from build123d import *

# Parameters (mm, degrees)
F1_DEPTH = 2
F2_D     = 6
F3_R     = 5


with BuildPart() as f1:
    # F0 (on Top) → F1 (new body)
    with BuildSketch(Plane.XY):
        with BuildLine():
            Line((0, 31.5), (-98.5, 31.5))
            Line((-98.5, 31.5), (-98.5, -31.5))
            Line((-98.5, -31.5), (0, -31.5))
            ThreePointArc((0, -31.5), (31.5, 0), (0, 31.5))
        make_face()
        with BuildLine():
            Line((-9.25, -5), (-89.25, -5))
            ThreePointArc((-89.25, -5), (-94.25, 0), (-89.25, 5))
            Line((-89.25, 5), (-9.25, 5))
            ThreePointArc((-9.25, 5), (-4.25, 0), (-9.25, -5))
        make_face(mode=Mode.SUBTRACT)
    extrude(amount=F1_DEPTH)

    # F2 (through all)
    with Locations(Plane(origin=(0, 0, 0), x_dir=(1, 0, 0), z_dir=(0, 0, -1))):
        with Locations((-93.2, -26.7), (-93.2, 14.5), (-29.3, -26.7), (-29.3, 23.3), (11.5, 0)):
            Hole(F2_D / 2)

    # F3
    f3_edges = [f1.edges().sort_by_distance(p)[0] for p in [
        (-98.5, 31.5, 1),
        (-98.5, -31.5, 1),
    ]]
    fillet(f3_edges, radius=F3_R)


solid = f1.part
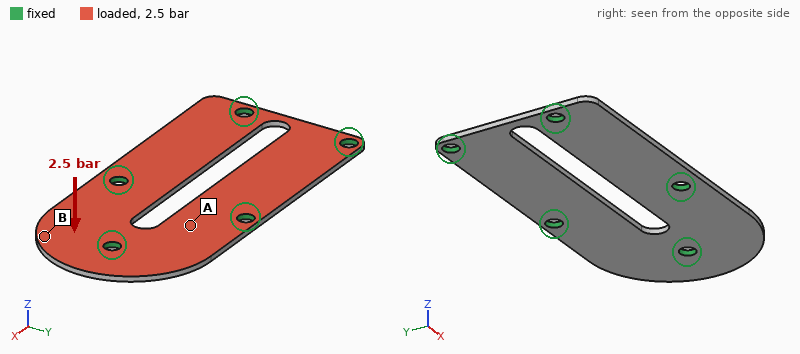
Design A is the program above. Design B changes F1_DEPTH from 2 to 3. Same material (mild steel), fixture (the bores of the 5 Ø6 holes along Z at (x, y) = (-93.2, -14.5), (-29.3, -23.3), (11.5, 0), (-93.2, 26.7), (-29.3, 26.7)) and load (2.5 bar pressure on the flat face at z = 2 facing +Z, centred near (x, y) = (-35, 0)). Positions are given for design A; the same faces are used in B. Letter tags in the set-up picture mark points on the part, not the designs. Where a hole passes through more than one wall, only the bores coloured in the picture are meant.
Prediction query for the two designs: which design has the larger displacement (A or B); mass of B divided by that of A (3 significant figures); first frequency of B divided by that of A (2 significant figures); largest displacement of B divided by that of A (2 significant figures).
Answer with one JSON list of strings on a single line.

["A", "1.50", "1.5", "0.31"]
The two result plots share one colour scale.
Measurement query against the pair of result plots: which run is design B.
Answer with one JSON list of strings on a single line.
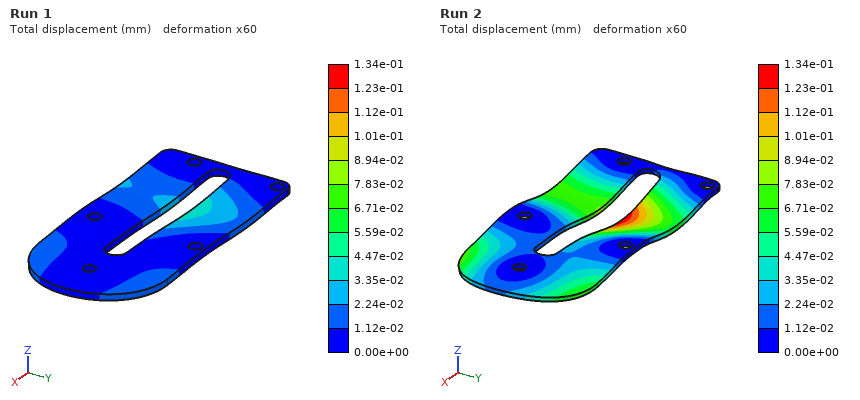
["Run 1"]
